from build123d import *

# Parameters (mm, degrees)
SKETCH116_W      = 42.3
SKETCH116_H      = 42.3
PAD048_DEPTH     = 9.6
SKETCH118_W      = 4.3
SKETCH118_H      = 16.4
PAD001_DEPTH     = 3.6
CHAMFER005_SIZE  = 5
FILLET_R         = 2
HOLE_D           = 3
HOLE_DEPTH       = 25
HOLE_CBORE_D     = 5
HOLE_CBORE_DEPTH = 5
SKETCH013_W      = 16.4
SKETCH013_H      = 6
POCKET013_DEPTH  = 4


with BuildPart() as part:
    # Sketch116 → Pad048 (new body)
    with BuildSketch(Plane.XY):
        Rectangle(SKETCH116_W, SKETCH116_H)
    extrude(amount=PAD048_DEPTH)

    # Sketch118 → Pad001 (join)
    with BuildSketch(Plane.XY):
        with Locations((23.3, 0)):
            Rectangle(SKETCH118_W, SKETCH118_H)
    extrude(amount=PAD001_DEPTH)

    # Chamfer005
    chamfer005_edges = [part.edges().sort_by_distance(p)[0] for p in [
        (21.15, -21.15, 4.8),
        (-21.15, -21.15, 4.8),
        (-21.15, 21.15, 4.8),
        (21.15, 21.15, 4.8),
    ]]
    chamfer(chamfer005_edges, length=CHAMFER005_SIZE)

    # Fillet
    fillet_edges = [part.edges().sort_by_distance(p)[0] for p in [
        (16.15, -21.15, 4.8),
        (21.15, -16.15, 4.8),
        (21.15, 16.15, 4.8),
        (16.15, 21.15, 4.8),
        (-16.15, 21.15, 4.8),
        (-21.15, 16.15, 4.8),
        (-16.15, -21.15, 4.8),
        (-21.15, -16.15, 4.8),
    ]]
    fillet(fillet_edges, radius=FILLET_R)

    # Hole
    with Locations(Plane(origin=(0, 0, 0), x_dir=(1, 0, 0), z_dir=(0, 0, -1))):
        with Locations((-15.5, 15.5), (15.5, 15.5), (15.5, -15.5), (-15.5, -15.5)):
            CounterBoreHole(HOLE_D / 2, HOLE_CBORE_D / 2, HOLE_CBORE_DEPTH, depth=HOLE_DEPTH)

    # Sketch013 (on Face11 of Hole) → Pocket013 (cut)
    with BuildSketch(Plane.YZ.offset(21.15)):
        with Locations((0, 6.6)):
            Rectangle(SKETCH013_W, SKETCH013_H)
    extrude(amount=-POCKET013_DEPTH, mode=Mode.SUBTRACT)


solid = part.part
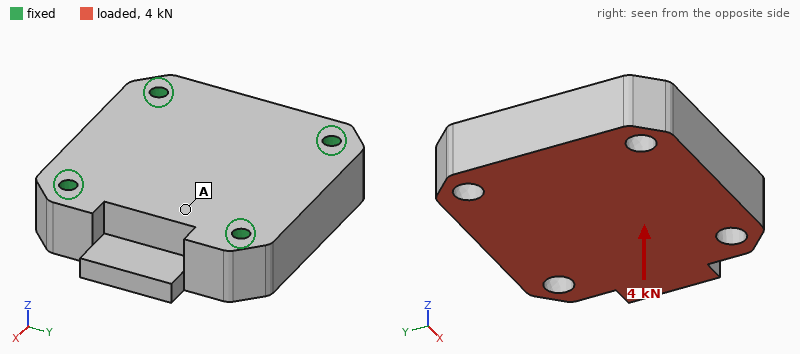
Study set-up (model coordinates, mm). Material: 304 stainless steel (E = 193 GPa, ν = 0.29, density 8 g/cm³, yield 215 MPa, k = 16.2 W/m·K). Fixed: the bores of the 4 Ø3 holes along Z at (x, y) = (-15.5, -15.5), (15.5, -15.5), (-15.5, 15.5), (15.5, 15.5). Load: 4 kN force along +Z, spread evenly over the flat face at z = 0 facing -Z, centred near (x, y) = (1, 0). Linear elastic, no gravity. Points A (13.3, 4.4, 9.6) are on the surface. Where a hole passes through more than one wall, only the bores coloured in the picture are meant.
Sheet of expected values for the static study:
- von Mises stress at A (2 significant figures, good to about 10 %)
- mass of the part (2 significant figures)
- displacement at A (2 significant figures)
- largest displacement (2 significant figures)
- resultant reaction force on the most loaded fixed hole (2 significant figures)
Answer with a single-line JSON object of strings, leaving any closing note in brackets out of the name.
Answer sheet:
{"von Mises stress at A": "11 MPa", "mass of the part": "130 g", "displacement at A": "2.2 µm", "largest displacement": "4.3 µm", "resultant reaction force on the most loaded fixed hole": "1.2 kN"}
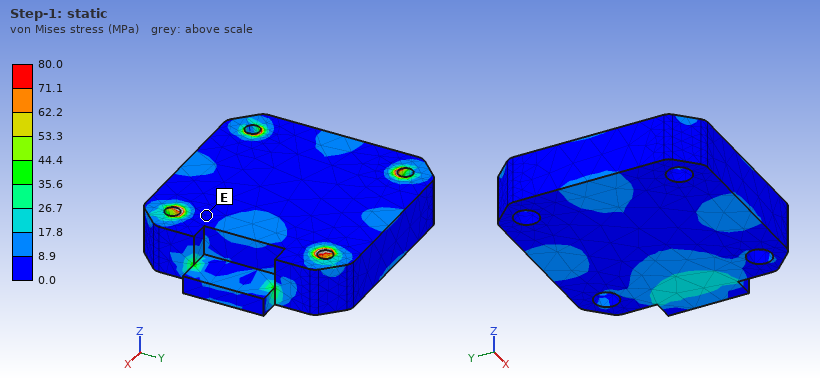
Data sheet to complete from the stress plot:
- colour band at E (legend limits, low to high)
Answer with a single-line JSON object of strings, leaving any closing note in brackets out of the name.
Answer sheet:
{"colour band at E": "0.0 to 8.9 MPa"}
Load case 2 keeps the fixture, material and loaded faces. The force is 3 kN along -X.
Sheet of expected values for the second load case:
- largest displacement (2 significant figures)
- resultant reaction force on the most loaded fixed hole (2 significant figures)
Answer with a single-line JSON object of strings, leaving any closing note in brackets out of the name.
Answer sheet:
{"largest displacement": "2.9 µm", "resultant reaction force on the most loaded fixed hole": "840 N"}
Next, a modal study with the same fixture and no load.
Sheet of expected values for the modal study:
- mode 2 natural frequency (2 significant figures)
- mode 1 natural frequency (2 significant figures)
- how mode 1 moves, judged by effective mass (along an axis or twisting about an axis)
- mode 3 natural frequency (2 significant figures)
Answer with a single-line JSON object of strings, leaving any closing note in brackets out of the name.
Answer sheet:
{"mode 2 natural frequency": "26 kHz", "mode 1 natural frequency": "20 kHz", "how mode 1 moves, judged by effective mass": "along Z", "mode 3 natural frequency": "28 kHz"}
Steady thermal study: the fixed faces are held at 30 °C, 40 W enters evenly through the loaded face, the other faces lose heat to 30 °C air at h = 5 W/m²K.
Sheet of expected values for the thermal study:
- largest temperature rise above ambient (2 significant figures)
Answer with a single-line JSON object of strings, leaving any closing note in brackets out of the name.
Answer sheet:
{"largest temperature rise above ambient": "63 K"}
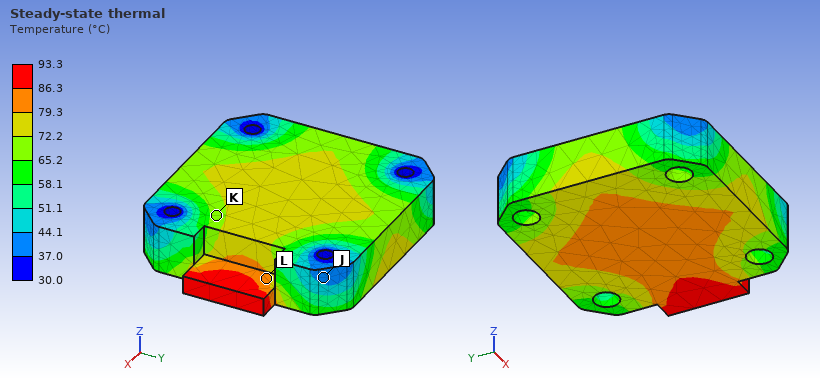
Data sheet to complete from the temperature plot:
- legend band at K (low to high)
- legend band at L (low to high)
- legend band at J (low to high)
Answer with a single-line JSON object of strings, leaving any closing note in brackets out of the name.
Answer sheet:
{"legend band at K": "65.2 to 72.2 °C", "legend band at L": "79.3 to 86.3 °C", "legend band at J": "37.0 to 44.1 °C"}
